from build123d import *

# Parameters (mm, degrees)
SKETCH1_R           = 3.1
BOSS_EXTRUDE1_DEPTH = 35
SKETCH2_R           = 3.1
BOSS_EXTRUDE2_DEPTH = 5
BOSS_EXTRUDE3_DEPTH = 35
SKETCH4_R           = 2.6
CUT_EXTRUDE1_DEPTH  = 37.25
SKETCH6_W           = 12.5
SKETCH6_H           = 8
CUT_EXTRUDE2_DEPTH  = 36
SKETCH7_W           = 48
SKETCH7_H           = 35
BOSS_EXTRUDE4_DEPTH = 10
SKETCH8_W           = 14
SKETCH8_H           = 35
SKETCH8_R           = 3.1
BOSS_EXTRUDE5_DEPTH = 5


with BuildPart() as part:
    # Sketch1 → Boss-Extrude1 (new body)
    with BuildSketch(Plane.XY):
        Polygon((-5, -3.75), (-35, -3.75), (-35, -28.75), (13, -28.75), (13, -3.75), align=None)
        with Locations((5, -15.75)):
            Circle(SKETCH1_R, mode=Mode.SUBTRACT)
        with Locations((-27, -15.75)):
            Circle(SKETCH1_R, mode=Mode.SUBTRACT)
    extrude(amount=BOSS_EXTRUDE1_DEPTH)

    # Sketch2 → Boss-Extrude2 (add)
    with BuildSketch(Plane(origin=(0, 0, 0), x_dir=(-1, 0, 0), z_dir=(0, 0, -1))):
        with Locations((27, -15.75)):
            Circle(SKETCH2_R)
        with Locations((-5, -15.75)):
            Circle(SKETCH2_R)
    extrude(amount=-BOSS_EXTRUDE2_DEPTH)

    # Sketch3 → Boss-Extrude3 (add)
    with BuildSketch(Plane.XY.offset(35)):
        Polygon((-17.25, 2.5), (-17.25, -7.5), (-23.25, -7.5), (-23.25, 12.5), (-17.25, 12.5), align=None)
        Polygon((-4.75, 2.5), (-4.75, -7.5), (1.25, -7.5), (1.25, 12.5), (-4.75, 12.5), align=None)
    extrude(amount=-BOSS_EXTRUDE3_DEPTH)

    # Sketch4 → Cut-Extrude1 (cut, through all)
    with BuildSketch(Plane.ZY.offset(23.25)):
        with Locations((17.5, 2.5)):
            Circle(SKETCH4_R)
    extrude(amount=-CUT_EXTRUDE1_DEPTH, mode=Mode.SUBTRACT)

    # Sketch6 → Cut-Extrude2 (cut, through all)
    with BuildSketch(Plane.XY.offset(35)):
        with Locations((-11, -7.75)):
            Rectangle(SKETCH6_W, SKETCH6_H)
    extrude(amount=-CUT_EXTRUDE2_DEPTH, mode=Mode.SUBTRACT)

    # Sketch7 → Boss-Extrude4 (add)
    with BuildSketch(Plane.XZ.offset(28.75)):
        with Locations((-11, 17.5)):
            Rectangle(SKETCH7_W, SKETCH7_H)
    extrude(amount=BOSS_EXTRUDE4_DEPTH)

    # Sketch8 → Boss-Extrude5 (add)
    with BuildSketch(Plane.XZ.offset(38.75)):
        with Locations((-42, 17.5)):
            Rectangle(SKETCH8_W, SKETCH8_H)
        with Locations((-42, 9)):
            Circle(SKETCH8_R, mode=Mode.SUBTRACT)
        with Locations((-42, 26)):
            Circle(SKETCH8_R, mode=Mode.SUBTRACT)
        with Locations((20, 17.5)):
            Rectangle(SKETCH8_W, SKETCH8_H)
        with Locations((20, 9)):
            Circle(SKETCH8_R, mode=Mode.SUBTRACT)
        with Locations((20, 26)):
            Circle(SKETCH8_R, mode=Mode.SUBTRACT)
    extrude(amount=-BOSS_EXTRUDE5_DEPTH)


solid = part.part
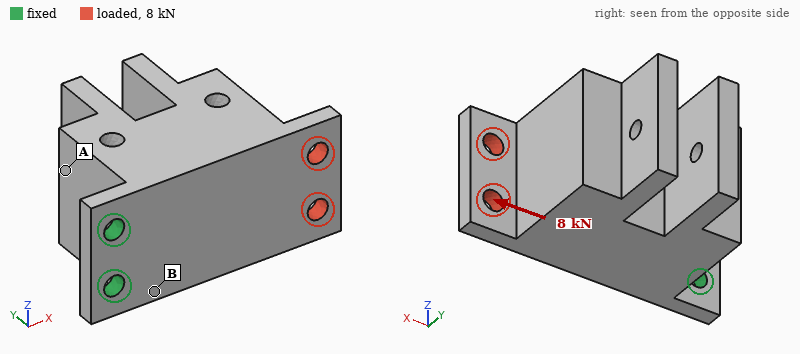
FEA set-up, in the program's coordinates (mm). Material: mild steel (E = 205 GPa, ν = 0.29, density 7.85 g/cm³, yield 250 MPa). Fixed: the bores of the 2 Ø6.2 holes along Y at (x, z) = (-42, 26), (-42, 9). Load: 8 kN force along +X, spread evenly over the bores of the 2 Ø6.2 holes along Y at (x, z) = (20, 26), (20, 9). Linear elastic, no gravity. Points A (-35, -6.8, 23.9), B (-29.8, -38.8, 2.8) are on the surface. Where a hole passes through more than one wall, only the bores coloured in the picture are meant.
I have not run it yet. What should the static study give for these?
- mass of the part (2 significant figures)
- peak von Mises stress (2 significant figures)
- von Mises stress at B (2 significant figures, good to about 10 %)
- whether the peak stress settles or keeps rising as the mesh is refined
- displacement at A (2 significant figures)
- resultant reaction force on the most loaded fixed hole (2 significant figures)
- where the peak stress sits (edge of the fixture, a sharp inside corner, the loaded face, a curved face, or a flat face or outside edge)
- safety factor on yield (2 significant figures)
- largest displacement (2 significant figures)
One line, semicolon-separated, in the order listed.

510 g; 120 MPa; 45 MPa; settles; 4.9 µm; 4.0 kN; the loaded face; 2.1; 32 µm
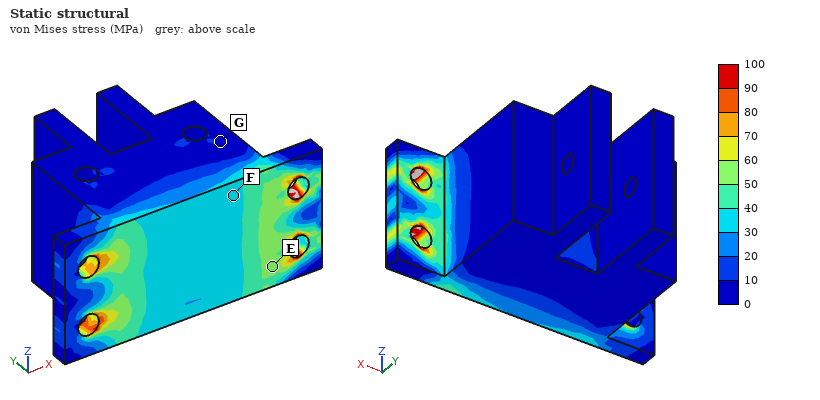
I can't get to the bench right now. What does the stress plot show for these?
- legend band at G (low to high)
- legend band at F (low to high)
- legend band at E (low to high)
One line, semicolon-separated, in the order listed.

0 to 10 MPa; 30 to 40 MPa; 50 to 60 MPa
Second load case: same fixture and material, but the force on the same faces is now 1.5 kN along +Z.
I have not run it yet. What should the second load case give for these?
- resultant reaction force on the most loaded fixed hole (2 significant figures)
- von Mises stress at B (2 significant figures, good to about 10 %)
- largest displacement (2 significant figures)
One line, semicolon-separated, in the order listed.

4.3 kN; 50 MPa; 38 µm
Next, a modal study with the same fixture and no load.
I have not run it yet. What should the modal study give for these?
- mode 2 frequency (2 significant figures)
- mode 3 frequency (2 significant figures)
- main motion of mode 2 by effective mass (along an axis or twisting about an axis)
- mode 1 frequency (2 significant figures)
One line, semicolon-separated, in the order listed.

2400 Hz; 3700 Hz; along Z; 600 Hz
